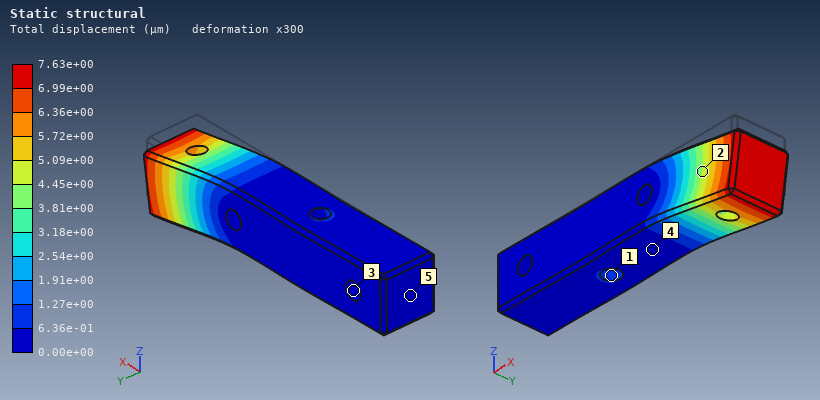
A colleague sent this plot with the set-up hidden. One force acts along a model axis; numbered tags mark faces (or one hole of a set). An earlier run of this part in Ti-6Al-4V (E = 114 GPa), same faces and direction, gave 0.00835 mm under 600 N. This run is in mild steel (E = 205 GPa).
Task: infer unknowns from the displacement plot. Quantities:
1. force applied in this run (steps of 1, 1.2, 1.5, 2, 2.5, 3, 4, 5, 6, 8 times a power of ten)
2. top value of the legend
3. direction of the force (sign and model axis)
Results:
1 kN
7.63e+00 µm
-Z
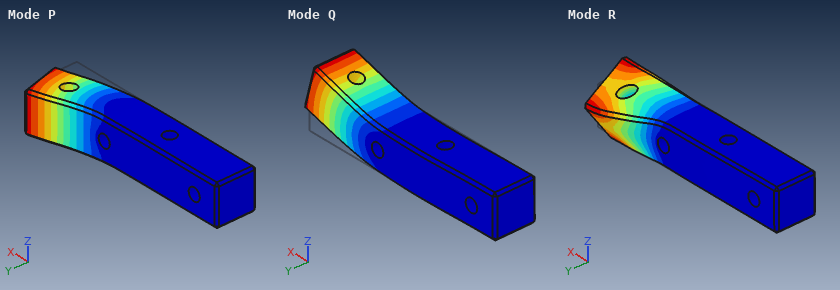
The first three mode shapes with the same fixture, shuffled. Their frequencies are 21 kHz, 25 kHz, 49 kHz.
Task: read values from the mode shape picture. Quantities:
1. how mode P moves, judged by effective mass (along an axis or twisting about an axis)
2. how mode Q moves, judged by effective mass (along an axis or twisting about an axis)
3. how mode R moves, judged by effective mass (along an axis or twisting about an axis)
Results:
along Y
along Z
twisting about X
